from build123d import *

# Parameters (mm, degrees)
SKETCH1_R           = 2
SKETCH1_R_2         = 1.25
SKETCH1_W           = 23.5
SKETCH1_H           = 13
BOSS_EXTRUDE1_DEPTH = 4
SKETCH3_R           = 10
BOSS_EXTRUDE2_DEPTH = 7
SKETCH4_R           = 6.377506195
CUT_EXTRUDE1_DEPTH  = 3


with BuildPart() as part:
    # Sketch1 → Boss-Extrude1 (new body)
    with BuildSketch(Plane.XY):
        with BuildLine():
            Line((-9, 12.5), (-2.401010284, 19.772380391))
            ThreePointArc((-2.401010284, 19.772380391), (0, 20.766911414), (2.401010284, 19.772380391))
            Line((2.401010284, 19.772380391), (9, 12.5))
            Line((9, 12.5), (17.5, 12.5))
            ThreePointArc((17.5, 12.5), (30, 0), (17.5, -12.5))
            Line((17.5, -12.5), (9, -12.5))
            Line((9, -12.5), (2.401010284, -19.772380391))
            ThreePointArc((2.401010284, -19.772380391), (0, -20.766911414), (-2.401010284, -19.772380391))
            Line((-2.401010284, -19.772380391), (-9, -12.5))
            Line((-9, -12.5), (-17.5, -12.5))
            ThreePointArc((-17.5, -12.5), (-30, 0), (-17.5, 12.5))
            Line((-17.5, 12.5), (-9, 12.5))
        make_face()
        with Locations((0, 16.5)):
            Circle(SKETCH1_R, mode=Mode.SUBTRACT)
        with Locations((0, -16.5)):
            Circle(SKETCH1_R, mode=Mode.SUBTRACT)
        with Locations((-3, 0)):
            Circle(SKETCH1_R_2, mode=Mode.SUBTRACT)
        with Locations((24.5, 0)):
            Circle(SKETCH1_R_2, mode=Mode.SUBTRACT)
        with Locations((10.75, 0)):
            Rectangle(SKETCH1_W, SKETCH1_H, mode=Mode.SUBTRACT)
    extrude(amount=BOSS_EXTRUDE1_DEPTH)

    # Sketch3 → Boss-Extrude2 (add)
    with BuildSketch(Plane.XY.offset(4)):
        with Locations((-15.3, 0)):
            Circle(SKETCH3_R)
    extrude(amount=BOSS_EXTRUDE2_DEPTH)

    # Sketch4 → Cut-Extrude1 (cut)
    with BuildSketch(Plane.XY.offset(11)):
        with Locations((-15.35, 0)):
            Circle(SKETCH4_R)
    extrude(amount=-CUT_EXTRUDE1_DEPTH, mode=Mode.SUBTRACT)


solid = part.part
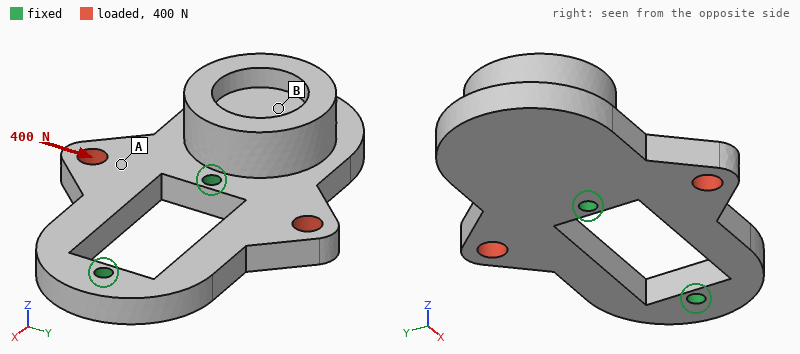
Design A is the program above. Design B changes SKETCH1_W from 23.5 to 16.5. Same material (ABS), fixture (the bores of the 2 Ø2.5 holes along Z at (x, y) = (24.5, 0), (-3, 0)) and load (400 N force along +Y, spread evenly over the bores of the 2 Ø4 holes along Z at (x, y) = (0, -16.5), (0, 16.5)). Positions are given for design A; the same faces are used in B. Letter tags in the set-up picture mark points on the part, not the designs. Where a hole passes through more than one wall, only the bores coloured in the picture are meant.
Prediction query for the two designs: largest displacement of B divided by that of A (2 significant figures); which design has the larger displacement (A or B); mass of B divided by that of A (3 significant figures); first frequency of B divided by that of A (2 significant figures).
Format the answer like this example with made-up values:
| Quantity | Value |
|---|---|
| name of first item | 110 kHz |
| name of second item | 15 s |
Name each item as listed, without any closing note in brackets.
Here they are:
| Quantity | Value |
|---|---|
| largest displacement of B divided by that of A | 0.65 |
| which design has the larger displacement | A |
| mass of B divided by that of A | 1.06 |
| first frequency of B divided by that of A | 1.0 |
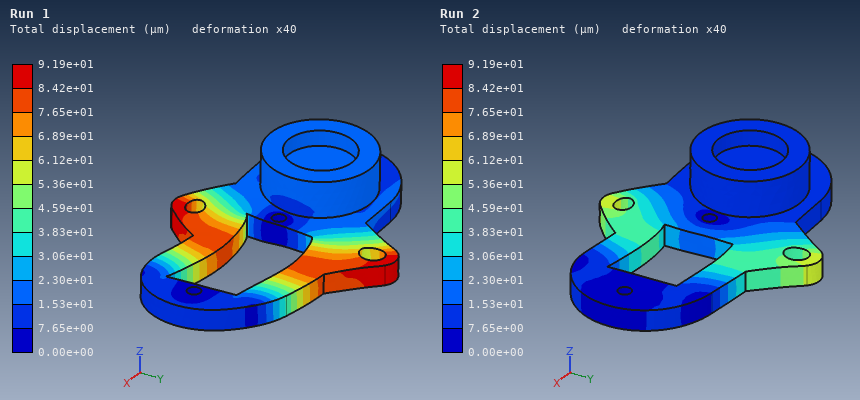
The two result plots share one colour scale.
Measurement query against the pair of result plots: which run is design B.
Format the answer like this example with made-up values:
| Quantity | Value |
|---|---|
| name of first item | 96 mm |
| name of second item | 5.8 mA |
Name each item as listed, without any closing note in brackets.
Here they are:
| Quantity | Value |
|---|---|
| which run is design B | Run 2 |
